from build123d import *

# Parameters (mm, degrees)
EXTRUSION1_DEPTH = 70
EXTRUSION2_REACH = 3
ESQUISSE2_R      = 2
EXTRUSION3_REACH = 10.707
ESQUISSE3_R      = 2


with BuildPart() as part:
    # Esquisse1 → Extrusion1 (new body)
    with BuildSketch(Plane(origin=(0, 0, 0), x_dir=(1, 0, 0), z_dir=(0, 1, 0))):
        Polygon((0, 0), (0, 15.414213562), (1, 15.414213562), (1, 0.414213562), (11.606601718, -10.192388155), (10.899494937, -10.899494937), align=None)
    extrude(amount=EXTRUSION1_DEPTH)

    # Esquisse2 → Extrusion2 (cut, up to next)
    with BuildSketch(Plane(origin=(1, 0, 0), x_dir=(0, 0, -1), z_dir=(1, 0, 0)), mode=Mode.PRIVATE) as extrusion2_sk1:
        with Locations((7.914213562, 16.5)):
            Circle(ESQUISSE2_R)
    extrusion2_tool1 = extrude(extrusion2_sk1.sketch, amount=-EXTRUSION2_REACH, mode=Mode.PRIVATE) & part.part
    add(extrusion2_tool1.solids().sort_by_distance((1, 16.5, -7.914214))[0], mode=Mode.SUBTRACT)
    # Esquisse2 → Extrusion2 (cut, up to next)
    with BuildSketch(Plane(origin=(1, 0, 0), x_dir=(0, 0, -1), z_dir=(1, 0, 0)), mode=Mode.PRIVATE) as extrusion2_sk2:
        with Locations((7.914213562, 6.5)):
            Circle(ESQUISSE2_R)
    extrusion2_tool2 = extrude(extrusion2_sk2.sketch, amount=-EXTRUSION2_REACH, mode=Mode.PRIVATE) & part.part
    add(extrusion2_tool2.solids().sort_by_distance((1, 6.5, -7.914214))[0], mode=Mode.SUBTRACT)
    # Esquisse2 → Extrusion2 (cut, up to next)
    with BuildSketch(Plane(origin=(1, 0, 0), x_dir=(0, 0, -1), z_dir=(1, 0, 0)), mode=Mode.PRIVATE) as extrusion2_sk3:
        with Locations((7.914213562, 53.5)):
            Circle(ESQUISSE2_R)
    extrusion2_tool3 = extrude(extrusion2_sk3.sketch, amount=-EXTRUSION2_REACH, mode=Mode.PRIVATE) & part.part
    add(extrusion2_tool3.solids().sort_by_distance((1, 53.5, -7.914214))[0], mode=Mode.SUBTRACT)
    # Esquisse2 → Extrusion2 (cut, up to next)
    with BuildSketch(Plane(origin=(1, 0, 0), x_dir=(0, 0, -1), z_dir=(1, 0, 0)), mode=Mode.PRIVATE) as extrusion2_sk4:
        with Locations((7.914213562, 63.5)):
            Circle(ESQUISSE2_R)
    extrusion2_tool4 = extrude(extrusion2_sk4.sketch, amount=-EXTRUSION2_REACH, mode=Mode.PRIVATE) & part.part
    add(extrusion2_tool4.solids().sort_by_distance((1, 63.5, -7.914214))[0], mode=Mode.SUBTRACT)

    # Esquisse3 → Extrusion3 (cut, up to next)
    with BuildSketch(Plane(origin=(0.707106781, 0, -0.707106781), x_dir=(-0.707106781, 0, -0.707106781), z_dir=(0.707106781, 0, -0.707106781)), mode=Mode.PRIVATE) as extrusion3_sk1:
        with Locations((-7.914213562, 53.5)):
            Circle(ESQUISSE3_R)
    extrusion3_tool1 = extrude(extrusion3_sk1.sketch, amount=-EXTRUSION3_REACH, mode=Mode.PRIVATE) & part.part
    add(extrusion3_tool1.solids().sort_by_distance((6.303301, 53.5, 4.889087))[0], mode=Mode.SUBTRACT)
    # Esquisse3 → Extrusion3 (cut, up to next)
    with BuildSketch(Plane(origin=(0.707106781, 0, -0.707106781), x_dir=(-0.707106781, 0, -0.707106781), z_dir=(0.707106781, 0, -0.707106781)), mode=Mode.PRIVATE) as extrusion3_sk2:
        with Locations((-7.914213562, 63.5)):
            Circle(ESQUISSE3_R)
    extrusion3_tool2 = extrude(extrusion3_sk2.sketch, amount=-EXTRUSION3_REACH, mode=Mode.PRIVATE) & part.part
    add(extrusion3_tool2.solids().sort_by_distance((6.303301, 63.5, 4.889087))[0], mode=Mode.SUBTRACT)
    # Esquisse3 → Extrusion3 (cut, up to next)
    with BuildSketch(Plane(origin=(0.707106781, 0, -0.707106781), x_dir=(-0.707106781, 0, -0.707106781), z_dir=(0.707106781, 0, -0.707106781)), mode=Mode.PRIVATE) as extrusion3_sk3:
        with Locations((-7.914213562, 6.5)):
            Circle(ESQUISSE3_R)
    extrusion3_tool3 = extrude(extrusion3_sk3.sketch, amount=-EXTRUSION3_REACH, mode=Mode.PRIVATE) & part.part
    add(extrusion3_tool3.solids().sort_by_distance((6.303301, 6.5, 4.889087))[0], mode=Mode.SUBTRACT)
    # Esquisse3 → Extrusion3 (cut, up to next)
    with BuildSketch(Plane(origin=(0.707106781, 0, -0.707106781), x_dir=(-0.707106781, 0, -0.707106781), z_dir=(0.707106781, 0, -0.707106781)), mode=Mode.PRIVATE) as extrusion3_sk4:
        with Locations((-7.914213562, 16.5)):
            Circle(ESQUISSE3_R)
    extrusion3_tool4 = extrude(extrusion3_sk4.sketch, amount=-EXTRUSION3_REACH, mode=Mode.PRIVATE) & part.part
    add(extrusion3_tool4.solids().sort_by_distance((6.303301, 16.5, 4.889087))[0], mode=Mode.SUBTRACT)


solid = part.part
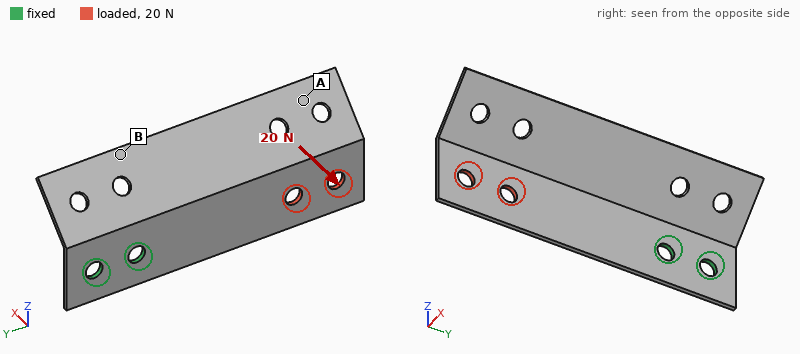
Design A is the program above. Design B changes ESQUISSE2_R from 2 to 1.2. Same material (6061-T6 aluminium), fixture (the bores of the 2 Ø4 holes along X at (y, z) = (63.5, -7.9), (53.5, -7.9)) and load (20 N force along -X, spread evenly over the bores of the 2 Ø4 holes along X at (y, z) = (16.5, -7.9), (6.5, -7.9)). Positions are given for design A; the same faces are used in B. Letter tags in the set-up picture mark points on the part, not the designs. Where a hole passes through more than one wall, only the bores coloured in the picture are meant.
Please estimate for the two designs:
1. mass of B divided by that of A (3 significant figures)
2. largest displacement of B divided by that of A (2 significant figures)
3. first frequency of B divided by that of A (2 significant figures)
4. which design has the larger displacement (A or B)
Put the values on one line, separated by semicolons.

1.02; 1.2; 0.87; B
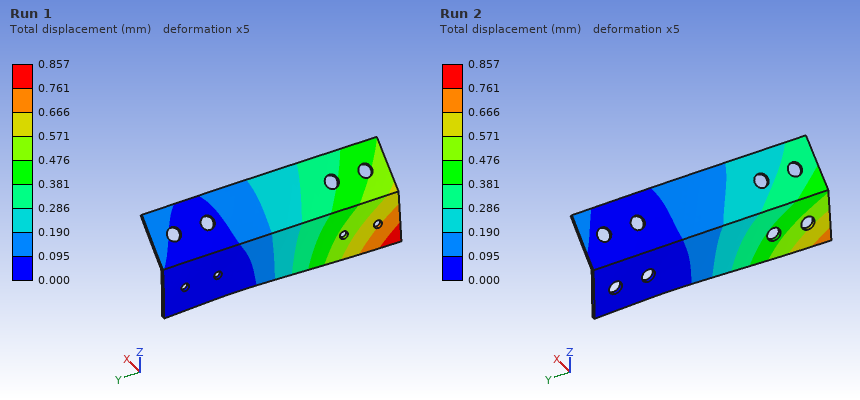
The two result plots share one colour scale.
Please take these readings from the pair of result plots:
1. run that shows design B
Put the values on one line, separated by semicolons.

Run 1
